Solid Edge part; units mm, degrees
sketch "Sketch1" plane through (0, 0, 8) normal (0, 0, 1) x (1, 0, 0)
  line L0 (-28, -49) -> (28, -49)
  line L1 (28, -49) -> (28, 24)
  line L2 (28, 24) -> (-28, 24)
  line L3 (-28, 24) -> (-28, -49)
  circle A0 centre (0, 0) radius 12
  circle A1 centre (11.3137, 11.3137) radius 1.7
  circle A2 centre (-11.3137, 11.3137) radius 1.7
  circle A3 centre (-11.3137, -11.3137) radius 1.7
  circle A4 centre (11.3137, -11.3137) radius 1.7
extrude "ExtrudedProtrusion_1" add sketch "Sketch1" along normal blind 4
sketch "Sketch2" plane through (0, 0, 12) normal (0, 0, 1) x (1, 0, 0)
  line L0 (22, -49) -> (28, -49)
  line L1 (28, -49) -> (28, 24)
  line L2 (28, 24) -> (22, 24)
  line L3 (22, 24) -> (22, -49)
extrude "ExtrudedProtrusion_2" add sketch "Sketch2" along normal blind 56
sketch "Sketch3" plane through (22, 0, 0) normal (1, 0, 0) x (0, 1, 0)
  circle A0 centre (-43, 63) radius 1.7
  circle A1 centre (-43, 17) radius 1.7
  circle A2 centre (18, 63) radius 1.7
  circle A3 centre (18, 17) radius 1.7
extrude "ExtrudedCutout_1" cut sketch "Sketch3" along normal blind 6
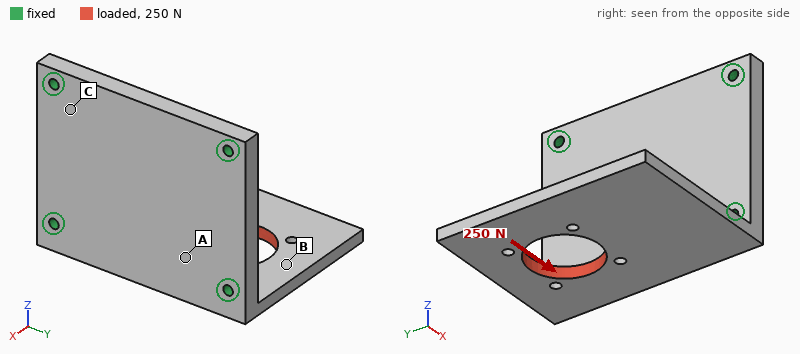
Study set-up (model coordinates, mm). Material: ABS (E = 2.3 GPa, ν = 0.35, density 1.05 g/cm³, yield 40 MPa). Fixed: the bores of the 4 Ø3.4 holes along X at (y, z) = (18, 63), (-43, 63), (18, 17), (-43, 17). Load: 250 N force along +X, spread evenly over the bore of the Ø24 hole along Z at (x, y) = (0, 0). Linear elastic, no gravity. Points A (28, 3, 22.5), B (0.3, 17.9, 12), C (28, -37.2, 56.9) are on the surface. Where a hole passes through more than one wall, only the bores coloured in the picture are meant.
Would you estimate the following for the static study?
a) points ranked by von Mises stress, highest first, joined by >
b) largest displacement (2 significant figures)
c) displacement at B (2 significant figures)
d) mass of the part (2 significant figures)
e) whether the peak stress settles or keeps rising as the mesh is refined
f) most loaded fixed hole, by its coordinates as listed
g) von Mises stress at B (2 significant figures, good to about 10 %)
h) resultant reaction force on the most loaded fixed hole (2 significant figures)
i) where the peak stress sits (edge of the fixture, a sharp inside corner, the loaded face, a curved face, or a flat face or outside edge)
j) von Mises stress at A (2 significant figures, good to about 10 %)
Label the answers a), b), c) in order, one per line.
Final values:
a) B > A > C
b) 0.29 mm
c) 0.15 mm
d) 41 g
e) keeps rising
f) (18, 17)
g) 2.4 MPa
h) 190 N
i) edge of the fixture
j) 1.2 MPa
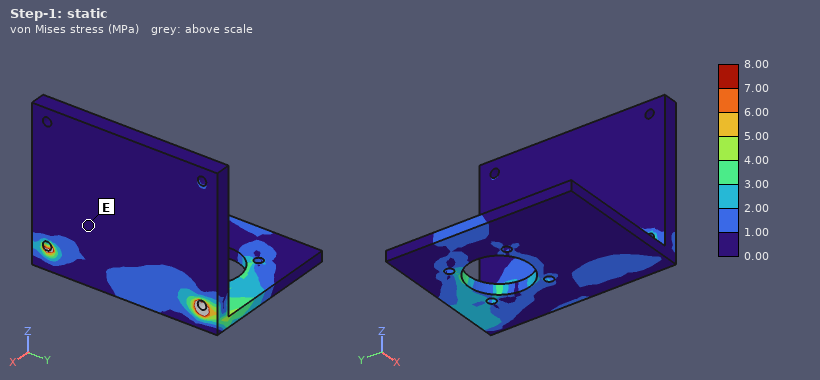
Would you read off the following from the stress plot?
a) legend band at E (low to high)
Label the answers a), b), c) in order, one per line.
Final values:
a) 0.00 to 1.00 MPa
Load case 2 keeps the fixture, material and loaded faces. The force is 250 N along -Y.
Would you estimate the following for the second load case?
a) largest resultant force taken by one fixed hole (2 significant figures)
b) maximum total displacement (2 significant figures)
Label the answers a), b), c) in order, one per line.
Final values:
a) 160 N
b) 0.17 mm
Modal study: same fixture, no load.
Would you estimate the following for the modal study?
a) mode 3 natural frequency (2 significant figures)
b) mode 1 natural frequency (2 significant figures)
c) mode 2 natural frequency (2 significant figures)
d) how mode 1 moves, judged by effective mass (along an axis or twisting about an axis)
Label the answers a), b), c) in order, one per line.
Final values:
a) 1500 Hz
b) 310 Hz
c) 600 Hz
d) along Z
